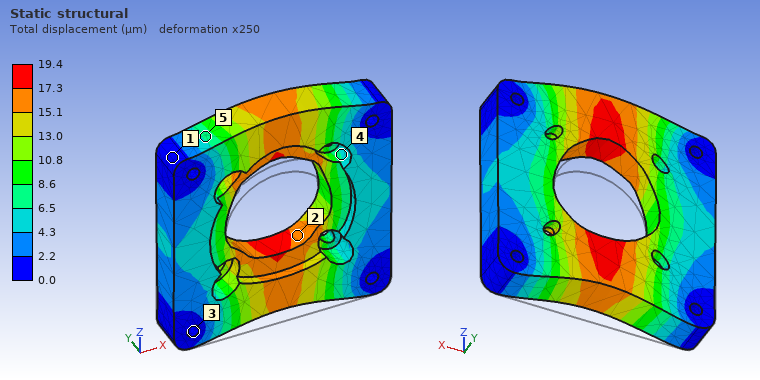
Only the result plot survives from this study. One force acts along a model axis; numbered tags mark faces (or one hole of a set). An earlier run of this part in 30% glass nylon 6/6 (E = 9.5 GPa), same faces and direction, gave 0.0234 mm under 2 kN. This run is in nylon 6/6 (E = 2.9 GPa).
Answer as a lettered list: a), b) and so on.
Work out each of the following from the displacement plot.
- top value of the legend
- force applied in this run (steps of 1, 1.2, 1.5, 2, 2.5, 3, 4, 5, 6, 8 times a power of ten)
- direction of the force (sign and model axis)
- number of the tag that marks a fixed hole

a) 19.4 µm
b) 500 N
c) +Z
d) 3
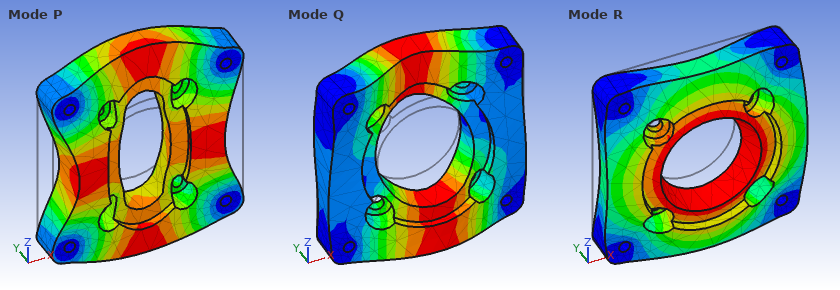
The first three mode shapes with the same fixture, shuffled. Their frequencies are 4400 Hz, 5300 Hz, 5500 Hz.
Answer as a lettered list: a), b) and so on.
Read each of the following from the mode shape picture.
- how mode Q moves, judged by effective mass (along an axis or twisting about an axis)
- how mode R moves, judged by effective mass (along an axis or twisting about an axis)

a) twisting about X
b) along Y
